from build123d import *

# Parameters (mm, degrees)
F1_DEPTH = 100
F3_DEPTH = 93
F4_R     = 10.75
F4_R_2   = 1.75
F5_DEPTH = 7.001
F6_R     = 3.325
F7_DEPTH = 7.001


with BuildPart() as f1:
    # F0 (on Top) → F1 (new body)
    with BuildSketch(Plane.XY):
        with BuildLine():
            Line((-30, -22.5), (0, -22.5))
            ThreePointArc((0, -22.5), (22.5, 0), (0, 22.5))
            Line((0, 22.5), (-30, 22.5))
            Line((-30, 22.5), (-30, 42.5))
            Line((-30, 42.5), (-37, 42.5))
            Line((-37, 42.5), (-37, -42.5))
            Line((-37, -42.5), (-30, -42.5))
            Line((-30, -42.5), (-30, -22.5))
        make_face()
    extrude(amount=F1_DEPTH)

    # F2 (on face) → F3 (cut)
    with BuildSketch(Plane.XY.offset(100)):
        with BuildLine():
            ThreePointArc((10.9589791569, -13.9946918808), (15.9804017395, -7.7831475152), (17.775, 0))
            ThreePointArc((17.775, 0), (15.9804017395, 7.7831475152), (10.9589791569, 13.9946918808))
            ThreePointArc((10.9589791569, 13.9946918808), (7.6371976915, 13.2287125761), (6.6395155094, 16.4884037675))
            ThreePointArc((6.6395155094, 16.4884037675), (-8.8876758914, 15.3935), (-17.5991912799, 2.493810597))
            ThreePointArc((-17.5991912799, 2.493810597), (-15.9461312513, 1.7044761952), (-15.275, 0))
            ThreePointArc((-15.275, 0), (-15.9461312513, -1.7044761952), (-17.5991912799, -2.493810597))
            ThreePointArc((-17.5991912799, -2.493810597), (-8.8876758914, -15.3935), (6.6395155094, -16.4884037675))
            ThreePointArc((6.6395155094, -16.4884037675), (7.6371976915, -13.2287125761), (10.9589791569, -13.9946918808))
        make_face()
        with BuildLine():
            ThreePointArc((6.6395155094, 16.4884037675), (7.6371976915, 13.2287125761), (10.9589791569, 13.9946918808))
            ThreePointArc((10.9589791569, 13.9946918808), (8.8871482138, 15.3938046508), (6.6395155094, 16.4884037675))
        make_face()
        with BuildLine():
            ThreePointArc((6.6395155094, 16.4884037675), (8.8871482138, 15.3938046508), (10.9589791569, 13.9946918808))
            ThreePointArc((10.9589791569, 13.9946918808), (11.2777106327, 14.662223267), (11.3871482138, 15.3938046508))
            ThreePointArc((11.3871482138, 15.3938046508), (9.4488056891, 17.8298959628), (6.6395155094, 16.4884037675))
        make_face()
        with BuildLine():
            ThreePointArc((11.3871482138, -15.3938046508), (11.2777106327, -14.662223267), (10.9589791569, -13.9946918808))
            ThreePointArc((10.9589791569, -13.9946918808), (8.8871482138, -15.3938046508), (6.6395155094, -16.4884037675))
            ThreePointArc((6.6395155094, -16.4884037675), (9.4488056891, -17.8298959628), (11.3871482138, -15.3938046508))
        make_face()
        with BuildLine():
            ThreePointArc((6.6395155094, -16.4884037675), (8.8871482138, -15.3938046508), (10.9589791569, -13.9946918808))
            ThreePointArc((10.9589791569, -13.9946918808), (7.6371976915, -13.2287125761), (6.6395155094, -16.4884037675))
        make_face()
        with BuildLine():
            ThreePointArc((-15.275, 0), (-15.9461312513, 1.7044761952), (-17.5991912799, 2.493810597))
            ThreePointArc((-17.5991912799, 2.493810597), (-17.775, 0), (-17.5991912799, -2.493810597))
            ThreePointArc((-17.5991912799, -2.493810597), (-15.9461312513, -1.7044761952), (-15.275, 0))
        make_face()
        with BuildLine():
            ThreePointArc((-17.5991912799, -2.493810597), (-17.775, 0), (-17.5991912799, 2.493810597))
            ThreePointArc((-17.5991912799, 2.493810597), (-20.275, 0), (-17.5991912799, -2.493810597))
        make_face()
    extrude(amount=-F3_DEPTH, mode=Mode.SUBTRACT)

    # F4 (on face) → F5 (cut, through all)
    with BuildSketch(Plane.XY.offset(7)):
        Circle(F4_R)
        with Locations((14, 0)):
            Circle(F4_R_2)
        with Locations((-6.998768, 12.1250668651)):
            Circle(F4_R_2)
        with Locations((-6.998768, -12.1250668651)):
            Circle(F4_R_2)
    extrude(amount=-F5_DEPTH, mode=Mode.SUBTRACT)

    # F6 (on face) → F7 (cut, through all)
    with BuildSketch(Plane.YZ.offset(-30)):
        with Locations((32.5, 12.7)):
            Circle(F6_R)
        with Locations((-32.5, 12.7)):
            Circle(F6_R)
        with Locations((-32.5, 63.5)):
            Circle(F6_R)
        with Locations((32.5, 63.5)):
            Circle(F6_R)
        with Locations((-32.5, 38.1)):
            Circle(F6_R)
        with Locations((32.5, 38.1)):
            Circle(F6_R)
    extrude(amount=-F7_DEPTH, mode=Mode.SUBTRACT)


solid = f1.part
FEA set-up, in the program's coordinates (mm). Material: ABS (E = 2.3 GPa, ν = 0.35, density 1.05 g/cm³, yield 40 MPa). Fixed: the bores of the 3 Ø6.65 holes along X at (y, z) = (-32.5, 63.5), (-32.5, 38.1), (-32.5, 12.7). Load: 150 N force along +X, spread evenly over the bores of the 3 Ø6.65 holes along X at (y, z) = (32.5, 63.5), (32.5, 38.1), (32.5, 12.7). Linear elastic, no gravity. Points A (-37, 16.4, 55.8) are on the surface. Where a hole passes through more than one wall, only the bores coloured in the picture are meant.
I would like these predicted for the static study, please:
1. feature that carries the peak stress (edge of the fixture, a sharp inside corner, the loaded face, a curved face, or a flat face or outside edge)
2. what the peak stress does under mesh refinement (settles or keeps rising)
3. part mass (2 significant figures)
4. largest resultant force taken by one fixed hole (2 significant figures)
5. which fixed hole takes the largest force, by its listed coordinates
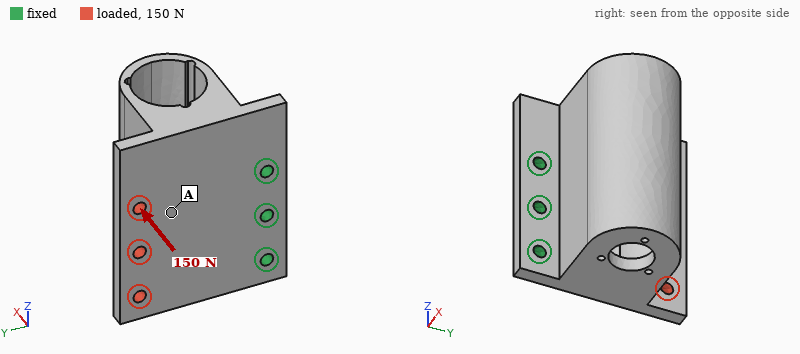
edge of the fixture
keeps rising
180 g
66 N
(-32.5, 38.1)
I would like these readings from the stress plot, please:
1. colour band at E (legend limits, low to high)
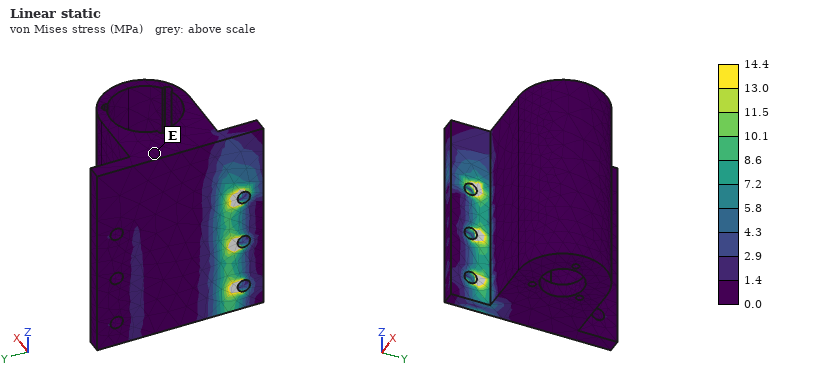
0.0 to 1.4 MPa
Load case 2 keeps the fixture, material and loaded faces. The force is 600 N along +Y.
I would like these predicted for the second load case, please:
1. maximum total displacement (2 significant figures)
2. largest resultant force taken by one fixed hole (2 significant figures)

70 µm
210 N
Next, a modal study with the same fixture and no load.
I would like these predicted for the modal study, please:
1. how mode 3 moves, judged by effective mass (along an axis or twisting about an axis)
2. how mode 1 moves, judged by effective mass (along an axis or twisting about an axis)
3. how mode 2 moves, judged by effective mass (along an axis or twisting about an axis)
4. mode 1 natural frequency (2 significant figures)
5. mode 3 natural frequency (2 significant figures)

along Z
along X
along Z
200 Hz
1100 Hz
